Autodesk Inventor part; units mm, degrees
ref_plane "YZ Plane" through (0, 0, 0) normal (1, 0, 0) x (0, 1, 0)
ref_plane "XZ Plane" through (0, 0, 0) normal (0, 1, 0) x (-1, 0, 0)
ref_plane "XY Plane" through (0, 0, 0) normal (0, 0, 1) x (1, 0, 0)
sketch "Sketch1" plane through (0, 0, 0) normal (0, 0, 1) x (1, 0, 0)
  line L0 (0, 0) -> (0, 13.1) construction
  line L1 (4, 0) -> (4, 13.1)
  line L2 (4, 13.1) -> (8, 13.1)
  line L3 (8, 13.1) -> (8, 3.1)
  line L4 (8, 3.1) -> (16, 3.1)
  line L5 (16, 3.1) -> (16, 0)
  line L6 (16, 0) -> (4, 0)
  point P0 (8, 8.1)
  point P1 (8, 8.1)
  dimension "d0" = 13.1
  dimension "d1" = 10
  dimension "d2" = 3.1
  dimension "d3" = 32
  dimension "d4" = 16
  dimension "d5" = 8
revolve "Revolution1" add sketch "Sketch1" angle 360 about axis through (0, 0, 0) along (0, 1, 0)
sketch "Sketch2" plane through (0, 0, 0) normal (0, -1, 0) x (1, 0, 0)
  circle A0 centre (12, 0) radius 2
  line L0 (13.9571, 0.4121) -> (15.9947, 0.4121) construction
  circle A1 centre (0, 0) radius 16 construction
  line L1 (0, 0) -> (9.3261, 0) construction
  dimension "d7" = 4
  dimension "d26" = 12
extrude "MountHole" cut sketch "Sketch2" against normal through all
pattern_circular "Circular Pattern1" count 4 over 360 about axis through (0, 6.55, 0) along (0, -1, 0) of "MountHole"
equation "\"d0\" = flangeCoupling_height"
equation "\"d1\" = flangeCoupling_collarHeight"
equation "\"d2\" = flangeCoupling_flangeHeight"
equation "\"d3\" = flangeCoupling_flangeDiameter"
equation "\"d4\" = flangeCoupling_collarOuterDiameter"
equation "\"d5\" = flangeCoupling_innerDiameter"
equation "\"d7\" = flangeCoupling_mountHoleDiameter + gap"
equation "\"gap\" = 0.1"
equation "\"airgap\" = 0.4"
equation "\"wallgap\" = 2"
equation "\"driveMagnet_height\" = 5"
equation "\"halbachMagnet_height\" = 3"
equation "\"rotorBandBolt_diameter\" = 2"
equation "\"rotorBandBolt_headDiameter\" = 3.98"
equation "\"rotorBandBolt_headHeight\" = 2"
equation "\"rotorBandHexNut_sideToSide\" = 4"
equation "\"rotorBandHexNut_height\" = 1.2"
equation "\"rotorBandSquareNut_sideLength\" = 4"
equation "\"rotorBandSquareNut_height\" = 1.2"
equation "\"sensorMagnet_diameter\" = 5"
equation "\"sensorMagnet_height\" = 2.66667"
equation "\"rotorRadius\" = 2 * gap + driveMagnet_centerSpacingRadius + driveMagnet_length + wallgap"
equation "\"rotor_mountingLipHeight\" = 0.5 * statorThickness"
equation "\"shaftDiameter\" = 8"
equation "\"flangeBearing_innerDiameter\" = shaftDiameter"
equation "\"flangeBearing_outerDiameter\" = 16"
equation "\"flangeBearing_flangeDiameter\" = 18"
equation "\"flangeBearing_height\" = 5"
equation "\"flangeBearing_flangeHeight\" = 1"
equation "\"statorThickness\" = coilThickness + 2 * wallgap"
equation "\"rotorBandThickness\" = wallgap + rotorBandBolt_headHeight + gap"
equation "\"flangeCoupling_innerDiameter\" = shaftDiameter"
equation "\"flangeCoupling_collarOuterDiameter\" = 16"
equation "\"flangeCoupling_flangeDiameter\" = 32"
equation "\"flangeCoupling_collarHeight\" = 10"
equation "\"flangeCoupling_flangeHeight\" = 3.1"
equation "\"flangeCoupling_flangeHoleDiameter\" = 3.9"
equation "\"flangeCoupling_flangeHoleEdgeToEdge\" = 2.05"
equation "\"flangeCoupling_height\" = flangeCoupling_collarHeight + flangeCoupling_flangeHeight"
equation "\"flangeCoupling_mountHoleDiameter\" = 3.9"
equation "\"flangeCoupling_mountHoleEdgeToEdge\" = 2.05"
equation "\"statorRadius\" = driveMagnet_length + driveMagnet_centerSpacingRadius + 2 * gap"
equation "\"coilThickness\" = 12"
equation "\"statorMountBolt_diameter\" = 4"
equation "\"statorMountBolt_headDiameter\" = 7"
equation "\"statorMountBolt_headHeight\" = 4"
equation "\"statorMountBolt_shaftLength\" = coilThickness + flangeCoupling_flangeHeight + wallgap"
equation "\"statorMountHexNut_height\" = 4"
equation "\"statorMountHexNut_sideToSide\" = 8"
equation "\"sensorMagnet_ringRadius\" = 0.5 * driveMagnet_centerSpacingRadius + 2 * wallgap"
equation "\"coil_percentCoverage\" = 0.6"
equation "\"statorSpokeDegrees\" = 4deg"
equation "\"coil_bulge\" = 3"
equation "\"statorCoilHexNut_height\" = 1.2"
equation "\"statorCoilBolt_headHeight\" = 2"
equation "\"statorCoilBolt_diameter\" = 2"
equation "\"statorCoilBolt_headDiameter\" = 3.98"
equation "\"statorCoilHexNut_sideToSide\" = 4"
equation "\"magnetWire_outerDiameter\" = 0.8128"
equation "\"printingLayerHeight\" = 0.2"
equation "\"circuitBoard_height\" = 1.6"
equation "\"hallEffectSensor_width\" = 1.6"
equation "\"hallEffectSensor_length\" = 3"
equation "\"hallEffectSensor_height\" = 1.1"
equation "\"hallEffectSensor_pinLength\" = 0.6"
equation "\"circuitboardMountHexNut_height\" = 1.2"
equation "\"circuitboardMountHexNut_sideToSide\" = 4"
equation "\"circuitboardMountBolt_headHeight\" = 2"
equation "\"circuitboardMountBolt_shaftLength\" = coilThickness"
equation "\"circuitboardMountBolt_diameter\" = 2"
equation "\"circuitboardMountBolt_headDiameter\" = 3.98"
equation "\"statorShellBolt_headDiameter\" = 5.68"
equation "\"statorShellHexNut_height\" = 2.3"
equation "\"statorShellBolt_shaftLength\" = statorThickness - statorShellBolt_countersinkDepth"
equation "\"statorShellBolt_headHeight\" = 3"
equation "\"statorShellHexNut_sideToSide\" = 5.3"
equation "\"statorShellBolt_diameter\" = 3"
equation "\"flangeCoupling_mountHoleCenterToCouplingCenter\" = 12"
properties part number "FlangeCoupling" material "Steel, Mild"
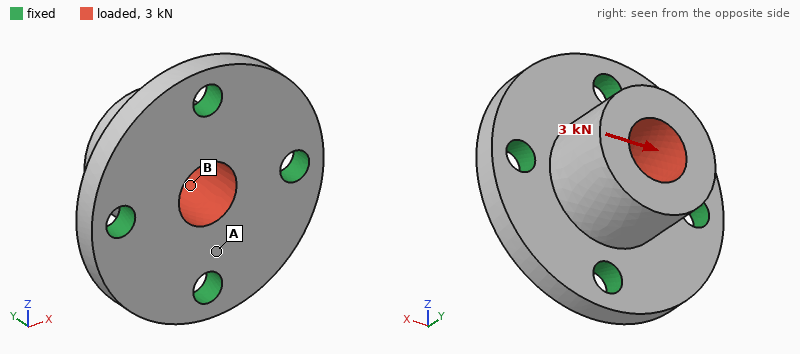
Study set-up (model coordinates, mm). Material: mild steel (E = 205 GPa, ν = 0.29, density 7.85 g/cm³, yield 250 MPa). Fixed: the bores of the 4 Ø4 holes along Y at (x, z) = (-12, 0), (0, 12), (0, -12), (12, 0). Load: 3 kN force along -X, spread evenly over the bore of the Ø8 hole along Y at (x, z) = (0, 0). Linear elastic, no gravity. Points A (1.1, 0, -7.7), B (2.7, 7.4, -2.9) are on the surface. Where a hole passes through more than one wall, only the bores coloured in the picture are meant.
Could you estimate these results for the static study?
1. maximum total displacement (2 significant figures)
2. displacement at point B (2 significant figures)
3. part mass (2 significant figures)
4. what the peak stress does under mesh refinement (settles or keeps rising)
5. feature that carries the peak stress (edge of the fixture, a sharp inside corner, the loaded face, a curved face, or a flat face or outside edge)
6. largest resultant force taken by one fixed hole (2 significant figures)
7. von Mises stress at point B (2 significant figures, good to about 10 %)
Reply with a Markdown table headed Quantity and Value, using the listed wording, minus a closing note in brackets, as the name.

| Quantity | Value |
|---|---|
| maximum total displacement | 6.1 µm |
| displacement at point B | 3.3 µm |
| part mass | 29 g |
| what the peak stress does under mesh refinement | keeps rising |
| feature that carries the peak stress | edge of the fixture |
| largest resultant force taken by one fixed hole | 1.2 kN |
| von Mises stress at point B | 30 MPa |
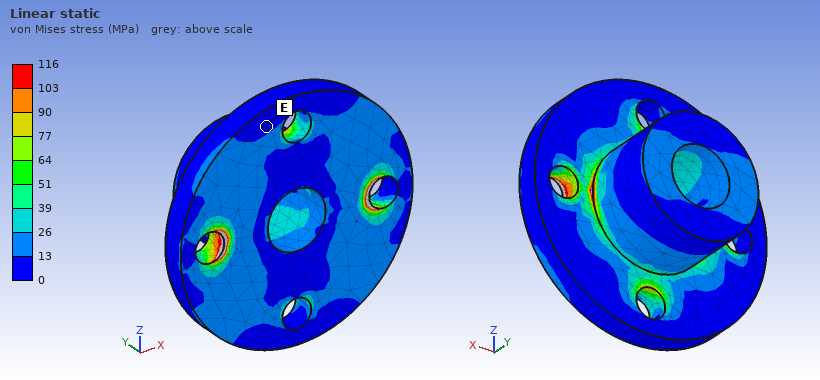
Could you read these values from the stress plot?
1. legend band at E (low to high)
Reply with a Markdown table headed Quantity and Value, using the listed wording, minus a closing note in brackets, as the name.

| Quantity | Value |
|---|---|
| legend band at E | 0 to 13 MPa |
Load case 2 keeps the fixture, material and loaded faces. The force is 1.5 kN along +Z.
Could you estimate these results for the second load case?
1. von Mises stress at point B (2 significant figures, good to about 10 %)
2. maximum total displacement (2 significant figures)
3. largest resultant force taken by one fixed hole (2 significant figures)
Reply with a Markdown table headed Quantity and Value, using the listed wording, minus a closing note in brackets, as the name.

| Quantity | Value |
|---|---|
| von Mises stress at point B | 14 MPa |
| maximum total displacement | 3.0 µm |
| largest resultant force taken by one fixed hole | 600 N |
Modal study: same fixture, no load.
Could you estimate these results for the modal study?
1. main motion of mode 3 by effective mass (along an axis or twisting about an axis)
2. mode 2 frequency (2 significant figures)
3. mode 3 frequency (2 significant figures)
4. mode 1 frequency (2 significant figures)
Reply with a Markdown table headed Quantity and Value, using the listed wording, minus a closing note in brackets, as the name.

| Quantity | Value |
|---|---|
| main motion of mode 3 by effective mass | along Y |
| mode 2 frequency | 32 kHz |
| mode 3 frequency | 39 kHz |
| mode 1 frequency | 32 kHz |
